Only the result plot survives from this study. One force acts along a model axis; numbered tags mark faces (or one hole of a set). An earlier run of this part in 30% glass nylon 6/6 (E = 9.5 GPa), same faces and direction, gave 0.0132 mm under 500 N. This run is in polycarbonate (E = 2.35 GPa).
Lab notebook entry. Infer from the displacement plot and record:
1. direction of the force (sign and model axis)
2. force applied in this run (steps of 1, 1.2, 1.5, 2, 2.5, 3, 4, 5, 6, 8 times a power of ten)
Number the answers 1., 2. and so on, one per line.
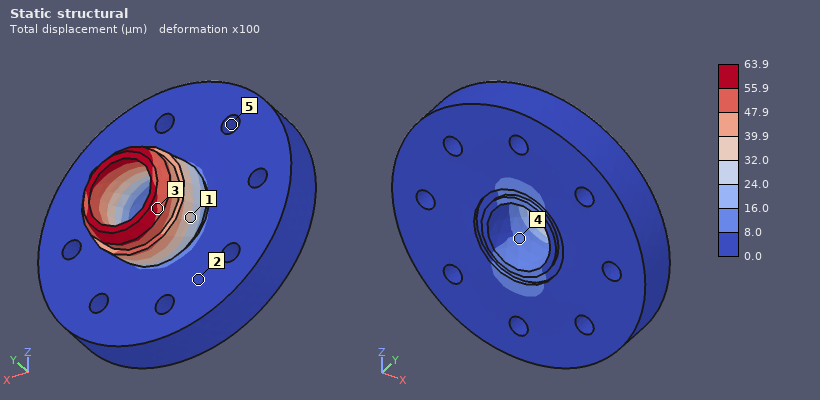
1. -Z
2. 600 N
